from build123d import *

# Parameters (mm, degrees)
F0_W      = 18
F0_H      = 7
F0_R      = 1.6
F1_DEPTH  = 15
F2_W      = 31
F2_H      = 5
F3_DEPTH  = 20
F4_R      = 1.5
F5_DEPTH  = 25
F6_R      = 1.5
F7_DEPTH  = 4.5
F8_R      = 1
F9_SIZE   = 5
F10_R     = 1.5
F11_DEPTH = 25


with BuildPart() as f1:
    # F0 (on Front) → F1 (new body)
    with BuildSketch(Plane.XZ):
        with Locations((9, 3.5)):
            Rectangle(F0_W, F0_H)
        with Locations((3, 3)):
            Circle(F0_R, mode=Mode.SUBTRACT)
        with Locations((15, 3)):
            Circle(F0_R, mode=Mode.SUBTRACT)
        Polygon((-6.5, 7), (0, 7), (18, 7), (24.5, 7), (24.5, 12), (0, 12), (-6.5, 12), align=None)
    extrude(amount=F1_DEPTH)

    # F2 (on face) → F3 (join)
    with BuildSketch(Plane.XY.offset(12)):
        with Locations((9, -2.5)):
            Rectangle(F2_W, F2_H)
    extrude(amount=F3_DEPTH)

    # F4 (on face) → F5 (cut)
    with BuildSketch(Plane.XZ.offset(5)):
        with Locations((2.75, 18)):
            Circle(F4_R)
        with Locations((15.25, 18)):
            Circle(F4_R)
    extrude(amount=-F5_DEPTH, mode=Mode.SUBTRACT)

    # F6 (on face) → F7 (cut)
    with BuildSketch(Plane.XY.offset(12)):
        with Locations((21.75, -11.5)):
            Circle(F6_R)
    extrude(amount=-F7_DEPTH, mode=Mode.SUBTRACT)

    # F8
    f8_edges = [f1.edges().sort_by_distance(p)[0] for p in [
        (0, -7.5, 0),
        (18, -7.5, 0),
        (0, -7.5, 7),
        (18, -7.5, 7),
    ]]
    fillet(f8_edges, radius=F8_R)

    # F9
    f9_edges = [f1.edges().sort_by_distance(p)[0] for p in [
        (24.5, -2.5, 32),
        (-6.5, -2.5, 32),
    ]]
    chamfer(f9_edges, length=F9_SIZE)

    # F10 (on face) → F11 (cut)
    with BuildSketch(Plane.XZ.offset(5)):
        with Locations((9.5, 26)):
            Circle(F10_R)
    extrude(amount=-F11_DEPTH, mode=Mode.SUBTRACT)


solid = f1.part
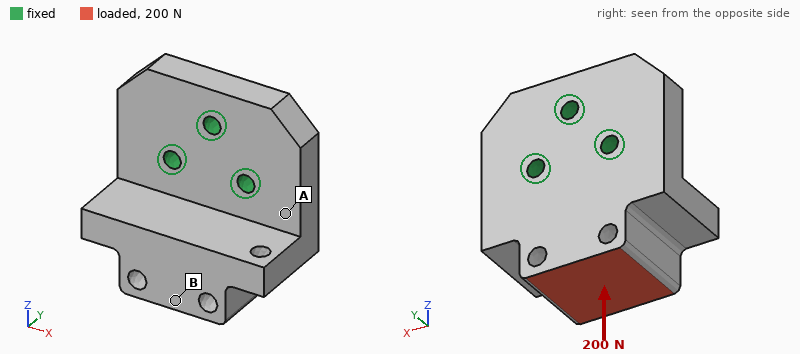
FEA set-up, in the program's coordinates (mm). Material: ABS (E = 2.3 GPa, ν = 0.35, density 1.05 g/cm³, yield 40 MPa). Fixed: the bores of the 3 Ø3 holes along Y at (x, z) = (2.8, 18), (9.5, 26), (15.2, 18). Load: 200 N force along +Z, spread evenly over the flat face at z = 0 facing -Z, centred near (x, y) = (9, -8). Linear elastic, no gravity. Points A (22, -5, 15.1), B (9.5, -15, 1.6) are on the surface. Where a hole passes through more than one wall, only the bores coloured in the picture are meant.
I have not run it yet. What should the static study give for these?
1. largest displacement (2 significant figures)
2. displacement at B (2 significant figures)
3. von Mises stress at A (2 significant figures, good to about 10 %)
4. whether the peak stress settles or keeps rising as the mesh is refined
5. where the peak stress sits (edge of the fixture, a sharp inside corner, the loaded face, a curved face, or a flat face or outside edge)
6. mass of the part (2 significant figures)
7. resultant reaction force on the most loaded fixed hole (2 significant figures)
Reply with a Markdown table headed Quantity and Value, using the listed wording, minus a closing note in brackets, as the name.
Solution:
| Quantity | Value |
|---|---|
| largest displacement | 0.24 mm |
| displacement at B | 0.22 mm |
| von Mises stress at A | 5.3 MPa |
| whether the peak stress settles or keeps rising as the mesh is refined | keeps rising |
| where the peak stress sits | edge of the fixture |
| mass of the part | 7.2 g |
| resultant reaction force on the most loaded fixed hole | 93 N |
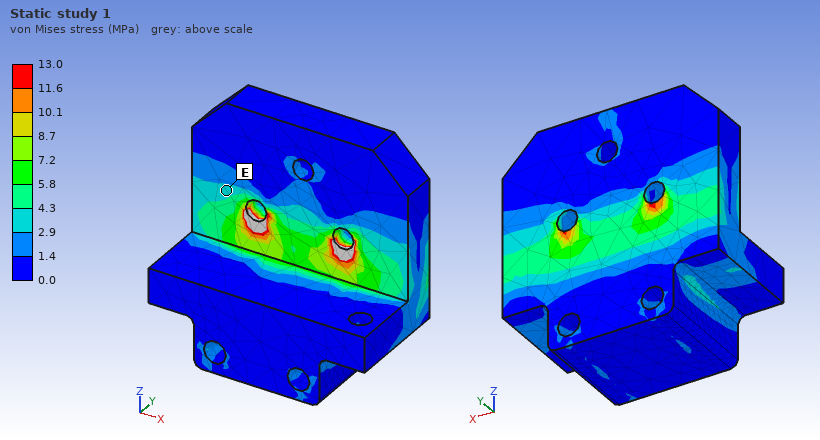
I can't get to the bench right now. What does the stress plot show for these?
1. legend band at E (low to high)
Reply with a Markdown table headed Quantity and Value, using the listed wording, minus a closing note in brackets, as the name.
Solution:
| Quantity | Value |
|---|---|
| legend band at E | 2.9 to 4.3 MPa |
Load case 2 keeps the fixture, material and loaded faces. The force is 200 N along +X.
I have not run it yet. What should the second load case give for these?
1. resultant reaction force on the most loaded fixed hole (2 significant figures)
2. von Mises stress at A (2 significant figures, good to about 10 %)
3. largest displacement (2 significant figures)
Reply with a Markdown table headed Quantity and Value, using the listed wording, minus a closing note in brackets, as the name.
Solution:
| Quantity | Value |
|---|---|
| resultant reaction force on the most loaded fixed hole | 250 N |
| von Mises stress at A | 3.1 MPa |
| largest displacement | 92 µm |
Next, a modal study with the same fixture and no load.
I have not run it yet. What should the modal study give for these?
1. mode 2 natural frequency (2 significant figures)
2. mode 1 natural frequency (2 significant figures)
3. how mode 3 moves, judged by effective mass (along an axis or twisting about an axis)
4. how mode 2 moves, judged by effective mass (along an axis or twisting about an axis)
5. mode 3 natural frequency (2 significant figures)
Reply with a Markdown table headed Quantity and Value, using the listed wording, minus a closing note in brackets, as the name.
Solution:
| Quantity | Value |
|---|---|
| mode 2 natural frequency | 4300 Hz |
| mode 1 natural frequency | 2100 Hz |
| how mode 3 moves, judged by effective mass | along X |
| how mode 2 moves, judged by effective mass | along X |
| mode 3 natural frequency | 6400 Hz |
